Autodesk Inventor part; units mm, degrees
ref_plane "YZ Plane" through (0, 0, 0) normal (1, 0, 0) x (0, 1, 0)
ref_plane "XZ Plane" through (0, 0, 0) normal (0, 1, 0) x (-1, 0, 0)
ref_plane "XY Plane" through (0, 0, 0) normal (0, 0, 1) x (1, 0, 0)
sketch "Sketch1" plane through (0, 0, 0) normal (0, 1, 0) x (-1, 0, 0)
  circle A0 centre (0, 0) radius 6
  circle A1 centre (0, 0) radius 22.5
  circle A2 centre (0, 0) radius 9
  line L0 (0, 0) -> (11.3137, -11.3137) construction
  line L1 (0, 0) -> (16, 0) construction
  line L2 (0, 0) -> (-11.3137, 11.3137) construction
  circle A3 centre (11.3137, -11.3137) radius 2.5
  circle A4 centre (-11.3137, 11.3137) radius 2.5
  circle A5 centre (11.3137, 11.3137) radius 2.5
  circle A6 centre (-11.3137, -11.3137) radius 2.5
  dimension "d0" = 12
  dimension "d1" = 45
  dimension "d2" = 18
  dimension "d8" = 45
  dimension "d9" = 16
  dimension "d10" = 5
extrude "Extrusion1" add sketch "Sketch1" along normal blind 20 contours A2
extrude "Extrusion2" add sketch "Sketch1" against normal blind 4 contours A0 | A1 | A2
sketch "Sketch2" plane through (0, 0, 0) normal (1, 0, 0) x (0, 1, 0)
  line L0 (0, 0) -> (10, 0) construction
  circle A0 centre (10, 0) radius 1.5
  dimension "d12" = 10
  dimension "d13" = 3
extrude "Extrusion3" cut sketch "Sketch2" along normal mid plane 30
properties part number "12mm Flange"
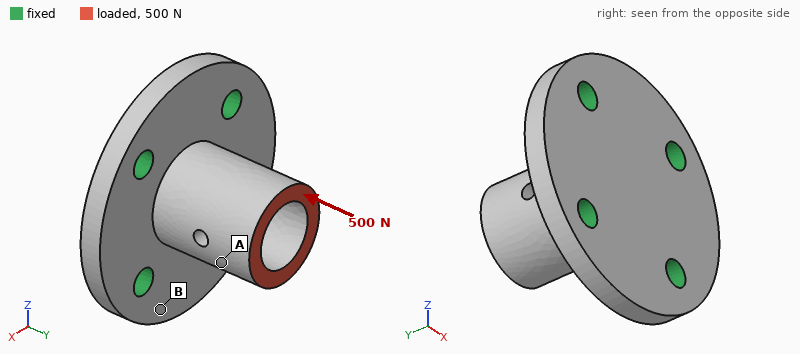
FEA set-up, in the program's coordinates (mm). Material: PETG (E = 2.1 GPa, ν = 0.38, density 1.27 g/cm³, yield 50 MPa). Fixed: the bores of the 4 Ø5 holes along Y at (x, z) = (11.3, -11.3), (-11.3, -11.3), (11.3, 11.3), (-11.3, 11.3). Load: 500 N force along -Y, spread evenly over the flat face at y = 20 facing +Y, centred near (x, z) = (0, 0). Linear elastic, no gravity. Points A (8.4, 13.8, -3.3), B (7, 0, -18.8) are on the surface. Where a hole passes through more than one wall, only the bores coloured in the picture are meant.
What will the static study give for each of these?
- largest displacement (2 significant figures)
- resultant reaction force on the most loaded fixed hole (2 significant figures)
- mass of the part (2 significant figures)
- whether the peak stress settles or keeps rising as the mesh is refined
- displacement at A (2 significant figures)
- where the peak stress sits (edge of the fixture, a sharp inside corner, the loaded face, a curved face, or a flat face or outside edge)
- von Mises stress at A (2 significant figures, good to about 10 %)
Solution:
91 µm
130 N
11 g
keeps rising
79 µm
edge of the fixture
4.3 MPa
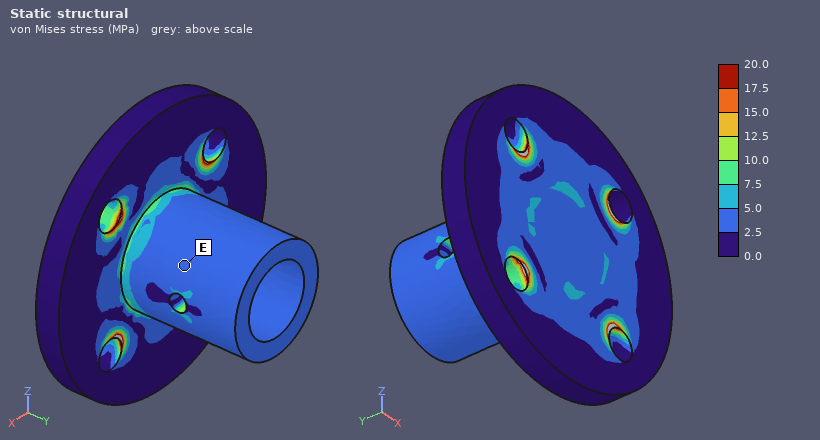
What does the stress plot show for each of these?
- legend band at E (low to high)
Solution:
2.5 to 5.0 MPa
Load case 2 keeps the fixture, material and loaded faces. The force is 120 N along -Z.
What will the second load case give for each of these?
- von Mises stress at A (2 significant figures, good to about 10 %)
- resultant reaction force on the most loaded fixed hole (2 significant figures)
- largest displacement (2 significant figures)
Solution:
2.1 MPa
76 N
0.18 mm
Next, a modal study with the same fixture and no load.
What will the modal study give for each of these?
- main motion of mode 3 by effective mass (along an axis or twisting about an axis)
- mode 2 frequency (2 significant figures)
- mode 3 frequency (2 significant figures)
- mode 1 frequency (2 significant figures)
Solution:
along Y
3800 Hz
6000 Hz
3700 Hz
